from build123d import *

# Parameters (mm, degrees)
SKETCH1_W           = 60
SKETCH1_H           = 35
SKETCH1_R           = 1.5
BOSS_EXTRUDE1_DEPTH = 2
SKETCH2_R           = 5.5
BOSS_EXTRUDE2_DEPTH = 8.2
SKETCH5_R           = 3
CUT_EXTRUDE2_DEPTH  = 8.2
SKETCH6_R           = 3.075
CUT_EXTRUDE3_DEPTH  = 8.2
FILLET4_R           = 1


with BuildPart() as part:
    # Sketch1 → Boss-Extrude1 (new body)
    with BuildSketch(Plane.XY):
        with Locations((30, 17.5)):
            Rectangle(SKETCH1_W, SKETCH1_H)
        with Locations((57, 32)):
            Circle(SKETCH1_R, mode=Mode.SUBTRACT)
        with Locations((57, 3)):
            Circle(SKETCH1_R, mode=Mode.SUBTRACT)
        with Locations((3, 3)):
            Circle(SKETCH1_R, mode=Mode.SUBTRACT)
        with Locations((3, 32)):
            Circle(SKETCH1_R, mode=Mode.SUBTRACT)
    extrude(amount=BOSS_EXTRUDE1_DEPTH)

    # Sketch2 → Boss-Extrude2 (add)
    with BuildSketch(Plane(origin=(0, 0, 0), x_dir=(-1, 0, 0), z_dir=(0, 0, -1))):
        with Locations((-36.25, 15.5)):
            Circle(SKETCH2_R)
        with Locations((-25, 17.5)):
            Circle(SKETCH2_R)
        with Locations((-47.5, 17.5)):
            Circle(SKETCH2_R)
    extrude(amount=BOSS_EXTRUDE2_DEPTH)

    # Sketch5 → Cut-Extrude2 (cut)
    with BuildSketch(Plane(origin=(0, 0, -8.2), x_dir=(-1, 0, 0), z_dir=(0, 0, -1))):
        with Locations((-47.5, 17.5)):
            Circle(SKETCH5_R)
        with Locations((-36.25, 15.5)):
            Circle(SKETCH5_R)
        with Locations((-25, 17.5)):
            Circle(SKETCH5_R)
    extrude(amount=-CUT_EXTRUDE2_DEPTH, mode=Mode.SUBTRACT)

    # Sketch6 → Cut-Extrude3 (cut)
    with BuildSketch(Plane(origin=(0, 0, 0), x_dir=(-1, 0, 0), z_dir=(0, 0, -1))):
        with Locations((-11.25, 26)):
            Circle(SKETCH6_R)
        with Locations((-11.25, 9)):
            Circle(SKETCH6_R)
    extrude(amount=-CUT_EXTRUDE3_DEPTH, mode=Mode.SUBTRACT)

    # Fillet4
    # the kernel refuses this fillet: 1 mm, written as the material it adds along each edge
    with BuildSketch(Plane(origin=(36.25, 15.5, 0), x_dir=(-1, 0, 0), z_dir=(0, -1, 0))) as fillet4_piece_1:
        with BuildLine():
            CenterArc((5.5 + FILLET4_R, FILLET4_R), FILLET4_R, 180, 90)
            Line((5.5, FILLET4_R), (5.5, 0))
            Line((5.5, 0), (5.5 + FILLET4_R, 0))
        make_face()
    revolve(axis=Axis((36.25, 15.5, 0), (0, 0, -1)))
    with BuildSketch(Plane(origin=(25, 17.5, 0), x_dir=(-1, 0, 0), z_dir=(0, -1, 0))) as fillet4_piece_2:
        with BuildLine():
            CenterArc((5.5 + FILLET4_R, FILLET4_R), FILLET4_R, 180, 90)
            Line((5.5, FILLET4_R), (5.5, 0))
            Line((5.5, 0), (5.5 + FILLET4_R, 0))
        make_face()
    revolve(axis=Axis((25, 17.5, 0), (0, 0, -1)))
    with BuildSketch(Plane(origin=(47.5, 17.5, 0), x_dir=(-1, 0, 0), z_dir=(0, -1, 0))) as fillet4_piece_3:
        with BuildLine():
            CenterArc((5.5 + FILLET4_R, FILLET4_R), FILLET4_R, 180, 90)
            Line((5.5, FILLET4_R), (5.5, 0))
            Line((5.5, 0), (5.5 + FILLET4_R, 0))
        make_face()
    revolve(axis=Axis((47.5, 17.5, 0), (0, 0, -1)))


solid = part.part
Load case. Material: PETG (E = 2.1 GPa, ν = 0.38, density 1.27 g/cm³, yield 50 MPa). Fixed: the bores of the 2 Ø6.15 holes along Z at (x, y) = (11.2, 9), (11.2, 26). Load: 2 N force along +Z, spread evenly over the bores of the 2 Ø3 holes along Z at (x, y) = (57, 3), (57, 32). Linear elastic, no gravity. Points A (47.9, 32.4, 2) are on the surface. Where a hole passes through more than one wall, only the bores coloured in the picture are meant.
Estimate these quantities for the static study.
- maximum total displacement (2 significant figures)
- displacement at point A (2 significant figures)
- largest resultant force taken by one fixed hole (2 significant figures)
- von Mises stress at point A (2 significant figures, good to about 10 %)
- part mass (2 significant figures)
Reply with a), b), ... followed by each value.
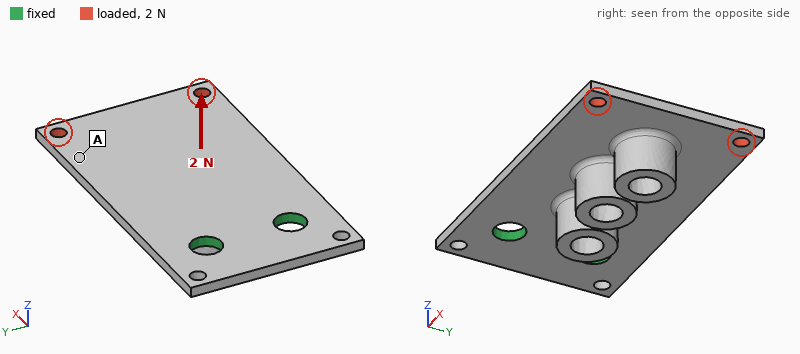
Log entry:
a) 0.82 mm
b) 0.52 mm
c) 1.2 N
d) 0.64 MPa
e) 7.2 g
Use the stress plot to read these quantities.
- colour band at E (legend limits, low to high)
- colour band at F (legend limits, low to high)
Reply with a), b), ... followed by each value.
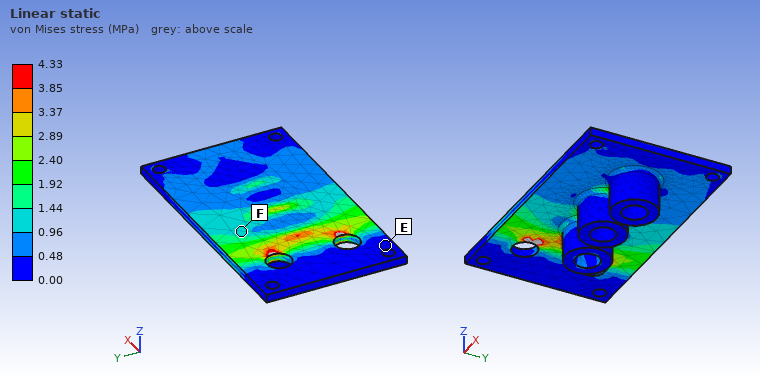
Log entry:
a) 0.00 to 0.48 MPa
b) 0.96 to 1.44 MPa
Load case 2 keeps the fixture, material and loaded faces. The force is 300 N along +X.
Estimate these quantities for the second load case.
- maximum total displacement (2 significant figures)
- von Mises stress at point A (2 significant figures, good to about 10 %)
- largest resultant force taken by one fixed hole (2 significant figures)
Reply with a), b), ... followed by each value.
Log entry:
a) 0.27 mm
b) 8.0 MPa
c) 150 N
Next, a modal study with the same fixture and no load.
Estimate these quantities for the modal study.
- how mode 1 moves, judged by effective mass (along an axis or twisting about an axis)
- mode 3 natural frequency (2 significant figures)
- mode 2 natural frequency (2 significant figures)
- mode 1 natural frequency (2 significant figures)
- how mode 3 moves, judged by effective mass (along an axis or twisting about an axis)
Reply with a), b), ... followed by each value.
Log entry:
a) along Z
b) 1200 Hz
c) 790 Hz
d) 200 Hz
e) along Z
